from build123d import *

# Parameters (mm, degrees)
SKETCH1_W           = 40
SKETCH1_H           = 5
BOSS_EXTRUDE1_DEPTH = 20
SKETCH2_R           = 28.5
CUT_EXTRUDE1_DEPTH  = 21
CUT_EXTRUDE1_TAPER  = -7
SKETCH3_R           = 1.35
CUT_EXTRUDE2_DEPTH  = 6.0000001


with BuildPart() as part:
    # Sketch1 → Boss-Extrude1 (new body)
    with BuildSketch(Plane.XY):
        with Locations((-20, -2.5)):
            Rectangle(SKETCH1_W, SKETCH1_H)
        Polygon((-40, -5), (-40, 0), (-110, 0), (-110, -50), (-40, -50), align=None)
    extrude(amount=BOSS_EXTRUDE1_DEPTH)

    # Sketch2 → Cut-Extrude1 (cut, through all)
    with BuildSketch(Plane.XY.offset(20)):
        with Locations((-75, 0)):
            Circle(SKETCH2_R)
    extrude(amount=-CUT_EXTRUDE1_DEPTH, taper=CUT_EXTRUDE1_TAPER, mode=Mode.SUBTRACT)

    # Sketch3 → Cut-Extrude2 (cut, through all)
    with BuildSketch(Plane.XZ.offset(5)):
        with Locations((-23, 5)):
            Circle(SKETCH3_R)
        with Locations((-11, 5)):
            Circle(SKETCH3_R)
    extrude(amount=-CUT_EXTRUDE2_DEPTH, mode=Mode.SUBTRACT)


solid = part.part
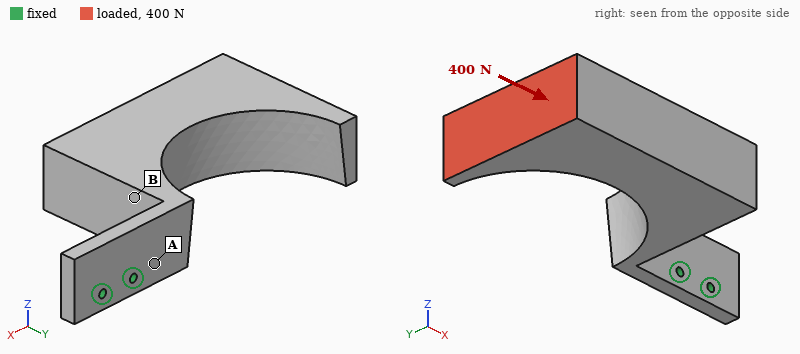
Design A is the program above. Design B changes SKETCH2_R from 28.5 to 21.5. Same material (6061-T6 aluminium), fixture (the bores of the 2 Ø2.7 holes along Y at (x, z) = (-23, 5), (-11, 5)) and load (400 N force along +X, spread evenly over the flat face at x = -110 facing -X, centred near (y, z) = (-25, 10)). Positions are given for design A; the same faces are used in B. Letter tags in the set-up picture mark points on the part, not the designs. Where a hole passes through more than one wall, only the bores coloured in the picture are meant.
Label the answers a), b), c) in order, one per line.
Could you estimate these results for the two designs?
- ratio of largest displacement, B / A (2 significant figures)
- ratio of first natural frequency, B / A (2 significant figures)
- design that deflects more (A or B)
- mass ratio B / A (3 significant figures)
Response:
a) 0.89
b) 0.98
c) A
d) 1.25
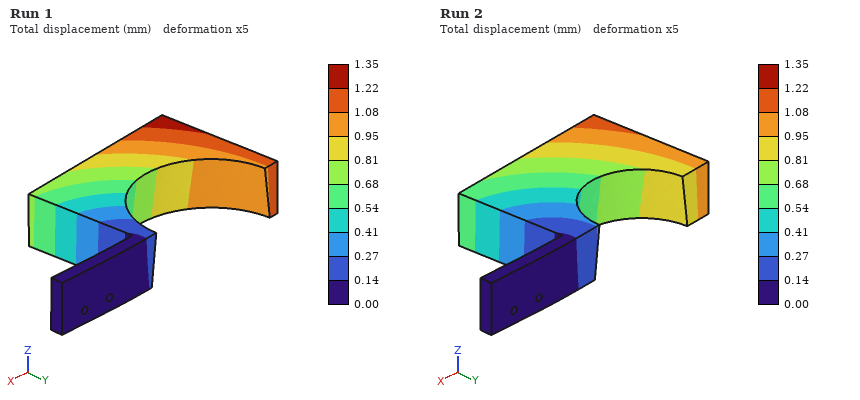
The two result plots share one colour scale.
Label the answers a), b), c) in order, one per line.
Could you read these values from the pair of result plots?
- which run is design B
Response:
a) Run 2
